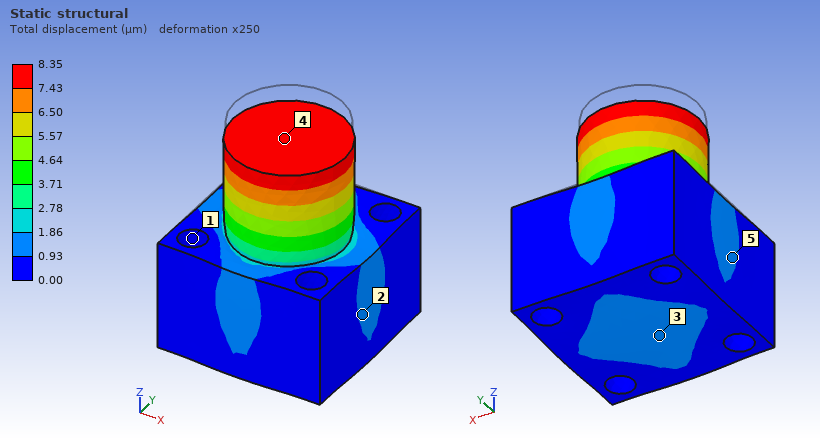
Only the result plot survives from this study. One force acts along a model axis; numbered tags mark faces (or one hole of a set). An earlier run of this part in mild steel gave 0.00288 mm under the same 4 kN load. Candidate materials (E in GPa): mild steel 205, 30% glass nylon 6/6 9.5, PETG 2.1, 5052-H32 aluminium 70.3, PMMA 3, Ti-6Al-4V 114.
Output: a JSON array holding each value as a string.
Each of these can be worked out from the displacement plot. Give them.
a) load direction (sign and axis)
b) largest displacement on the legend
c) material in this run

["-Z", "8.35 µm", "5052-H32 aluminium"]
